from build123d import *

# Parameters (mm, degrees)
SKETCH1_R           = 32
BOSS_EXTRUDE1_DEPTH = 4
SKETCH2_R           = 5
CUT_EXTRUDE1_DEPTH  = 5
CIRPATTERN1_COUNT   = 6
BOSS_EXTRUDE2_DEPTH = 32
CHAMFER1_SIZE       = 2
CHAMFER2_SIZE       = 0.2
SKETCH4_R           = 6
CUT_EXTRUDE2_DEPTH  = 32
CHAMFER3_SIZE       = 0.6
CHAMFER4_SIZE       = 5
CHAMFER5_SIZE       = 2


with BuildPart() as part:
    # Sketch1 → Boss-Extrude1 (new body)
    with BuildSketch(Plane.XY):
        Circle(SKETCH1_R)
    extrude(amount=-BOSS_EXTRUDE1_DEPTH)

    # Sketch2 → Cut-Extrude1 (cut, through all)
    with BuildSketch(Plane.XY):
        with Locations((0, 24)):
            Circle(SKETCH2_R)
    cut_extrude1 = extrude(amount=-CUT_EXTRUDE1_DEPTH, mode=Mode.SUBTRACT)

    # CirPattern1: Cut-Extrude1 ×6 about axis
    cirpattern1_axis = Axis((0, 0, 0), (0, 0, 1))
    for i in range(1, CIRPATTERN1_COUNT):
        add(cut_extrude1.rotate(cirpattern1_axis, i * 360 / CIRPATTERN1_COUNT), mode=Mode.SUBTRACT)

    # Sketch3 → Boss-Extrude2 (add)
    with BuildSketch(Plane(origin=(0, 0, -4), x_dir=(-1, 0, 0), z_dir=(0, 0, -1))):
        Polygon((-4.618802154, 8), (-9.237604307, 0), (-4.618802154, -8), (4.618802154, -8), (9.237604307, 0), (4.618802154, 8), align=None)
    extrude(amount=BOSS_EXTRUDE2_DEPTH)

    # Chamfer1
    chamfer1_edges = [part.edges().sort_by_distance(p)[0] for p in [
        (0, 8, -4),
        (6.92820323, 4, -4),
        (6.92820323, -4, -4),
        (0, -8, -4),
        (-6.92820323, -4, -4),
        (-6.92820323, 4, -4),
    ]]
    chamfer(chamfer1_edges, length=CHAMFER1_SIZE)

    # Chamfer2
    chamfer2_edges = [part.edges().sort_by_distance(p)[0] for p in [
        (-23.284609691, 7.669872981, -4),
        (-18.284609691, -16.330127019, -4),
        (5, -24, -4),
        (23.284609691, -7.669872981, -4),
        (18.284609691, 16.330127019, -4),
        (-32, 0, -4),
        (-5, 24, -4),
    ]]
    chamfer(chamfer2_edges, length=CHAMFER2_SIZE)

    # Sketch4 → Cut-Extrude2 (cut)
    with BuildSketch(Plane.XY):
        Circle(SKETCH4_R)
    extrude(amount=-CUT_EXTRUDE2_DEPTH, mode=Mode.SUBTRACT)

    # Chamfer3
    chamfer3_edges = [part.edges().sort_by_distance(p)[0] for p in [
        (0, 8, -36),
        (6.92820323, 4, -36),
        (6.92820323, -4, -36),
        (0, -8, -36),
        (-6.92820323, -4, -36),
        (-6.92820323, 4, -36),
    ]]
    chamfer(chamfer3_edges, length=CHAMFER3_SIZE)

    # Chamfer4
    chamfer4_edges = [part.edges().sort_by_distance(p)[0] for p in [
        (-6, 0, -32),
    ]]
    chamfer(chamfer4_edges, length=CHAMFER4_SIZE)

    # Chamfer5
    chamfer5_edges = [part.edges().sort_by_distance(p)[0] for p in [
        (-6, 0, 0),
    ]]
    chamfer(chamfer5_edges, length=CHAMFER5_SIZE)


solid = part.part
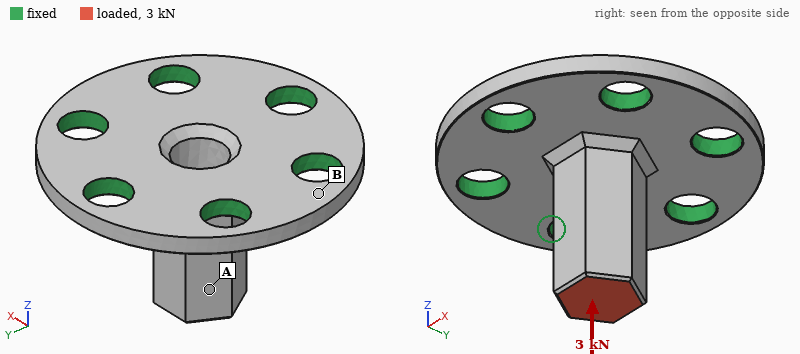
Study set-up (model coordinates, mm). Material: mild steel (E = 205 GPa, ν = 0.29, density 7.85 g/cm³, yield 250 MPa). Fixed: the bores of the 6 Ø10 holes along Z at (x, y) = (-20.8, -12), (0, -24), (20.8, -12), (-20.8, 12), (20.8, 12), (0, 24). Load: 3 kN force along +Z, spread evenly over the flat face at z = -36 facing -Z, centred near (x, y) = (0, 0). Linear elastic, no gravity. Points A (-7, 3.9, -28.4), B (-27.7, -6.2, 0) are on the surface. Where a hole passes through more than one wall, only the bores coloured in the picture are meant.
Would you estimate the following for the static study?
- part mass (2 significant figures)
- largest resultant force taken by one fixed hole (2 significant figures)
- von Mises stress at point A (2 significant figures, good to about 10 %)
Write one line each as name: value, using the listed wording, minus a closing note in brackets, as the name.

part mass: 120 g
largest resultant force taken by one fixed hole: 640 N
von Mises stress at point A: 24 MPa
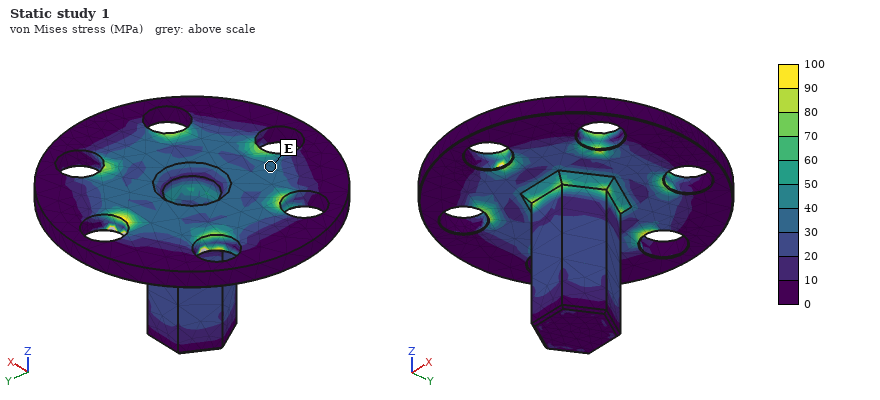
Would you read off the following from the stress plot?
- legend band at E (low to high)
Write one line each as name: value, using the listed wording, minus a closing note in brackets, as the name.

legend band at E: 30 to 40 MPa
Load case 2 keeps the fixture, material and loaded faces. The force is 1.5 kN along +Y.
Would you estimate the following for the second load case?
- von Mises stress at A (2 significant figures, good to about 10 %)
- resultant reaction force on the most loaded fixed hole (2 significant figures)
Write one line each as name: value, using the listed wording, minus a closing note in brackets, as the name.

von Mises stress at A: 34 MPa
resultant reaction force on the most loaded fixed hole: 1.2 kN
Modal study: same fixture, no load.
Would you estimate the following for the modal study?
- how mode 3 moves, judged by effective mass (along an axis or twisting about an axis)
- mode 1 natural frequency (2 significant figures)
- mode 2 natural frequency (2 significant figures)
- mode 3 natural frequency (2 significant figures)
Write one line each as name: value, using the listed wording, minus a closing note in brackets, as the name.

how mode 3 moves, judged by effective mass: along Z
mode 1 natural frequency: 6000 Hz
mode 2 natural frequency: 6000 Hz
mode 3 natural frequency: 14 kHz
